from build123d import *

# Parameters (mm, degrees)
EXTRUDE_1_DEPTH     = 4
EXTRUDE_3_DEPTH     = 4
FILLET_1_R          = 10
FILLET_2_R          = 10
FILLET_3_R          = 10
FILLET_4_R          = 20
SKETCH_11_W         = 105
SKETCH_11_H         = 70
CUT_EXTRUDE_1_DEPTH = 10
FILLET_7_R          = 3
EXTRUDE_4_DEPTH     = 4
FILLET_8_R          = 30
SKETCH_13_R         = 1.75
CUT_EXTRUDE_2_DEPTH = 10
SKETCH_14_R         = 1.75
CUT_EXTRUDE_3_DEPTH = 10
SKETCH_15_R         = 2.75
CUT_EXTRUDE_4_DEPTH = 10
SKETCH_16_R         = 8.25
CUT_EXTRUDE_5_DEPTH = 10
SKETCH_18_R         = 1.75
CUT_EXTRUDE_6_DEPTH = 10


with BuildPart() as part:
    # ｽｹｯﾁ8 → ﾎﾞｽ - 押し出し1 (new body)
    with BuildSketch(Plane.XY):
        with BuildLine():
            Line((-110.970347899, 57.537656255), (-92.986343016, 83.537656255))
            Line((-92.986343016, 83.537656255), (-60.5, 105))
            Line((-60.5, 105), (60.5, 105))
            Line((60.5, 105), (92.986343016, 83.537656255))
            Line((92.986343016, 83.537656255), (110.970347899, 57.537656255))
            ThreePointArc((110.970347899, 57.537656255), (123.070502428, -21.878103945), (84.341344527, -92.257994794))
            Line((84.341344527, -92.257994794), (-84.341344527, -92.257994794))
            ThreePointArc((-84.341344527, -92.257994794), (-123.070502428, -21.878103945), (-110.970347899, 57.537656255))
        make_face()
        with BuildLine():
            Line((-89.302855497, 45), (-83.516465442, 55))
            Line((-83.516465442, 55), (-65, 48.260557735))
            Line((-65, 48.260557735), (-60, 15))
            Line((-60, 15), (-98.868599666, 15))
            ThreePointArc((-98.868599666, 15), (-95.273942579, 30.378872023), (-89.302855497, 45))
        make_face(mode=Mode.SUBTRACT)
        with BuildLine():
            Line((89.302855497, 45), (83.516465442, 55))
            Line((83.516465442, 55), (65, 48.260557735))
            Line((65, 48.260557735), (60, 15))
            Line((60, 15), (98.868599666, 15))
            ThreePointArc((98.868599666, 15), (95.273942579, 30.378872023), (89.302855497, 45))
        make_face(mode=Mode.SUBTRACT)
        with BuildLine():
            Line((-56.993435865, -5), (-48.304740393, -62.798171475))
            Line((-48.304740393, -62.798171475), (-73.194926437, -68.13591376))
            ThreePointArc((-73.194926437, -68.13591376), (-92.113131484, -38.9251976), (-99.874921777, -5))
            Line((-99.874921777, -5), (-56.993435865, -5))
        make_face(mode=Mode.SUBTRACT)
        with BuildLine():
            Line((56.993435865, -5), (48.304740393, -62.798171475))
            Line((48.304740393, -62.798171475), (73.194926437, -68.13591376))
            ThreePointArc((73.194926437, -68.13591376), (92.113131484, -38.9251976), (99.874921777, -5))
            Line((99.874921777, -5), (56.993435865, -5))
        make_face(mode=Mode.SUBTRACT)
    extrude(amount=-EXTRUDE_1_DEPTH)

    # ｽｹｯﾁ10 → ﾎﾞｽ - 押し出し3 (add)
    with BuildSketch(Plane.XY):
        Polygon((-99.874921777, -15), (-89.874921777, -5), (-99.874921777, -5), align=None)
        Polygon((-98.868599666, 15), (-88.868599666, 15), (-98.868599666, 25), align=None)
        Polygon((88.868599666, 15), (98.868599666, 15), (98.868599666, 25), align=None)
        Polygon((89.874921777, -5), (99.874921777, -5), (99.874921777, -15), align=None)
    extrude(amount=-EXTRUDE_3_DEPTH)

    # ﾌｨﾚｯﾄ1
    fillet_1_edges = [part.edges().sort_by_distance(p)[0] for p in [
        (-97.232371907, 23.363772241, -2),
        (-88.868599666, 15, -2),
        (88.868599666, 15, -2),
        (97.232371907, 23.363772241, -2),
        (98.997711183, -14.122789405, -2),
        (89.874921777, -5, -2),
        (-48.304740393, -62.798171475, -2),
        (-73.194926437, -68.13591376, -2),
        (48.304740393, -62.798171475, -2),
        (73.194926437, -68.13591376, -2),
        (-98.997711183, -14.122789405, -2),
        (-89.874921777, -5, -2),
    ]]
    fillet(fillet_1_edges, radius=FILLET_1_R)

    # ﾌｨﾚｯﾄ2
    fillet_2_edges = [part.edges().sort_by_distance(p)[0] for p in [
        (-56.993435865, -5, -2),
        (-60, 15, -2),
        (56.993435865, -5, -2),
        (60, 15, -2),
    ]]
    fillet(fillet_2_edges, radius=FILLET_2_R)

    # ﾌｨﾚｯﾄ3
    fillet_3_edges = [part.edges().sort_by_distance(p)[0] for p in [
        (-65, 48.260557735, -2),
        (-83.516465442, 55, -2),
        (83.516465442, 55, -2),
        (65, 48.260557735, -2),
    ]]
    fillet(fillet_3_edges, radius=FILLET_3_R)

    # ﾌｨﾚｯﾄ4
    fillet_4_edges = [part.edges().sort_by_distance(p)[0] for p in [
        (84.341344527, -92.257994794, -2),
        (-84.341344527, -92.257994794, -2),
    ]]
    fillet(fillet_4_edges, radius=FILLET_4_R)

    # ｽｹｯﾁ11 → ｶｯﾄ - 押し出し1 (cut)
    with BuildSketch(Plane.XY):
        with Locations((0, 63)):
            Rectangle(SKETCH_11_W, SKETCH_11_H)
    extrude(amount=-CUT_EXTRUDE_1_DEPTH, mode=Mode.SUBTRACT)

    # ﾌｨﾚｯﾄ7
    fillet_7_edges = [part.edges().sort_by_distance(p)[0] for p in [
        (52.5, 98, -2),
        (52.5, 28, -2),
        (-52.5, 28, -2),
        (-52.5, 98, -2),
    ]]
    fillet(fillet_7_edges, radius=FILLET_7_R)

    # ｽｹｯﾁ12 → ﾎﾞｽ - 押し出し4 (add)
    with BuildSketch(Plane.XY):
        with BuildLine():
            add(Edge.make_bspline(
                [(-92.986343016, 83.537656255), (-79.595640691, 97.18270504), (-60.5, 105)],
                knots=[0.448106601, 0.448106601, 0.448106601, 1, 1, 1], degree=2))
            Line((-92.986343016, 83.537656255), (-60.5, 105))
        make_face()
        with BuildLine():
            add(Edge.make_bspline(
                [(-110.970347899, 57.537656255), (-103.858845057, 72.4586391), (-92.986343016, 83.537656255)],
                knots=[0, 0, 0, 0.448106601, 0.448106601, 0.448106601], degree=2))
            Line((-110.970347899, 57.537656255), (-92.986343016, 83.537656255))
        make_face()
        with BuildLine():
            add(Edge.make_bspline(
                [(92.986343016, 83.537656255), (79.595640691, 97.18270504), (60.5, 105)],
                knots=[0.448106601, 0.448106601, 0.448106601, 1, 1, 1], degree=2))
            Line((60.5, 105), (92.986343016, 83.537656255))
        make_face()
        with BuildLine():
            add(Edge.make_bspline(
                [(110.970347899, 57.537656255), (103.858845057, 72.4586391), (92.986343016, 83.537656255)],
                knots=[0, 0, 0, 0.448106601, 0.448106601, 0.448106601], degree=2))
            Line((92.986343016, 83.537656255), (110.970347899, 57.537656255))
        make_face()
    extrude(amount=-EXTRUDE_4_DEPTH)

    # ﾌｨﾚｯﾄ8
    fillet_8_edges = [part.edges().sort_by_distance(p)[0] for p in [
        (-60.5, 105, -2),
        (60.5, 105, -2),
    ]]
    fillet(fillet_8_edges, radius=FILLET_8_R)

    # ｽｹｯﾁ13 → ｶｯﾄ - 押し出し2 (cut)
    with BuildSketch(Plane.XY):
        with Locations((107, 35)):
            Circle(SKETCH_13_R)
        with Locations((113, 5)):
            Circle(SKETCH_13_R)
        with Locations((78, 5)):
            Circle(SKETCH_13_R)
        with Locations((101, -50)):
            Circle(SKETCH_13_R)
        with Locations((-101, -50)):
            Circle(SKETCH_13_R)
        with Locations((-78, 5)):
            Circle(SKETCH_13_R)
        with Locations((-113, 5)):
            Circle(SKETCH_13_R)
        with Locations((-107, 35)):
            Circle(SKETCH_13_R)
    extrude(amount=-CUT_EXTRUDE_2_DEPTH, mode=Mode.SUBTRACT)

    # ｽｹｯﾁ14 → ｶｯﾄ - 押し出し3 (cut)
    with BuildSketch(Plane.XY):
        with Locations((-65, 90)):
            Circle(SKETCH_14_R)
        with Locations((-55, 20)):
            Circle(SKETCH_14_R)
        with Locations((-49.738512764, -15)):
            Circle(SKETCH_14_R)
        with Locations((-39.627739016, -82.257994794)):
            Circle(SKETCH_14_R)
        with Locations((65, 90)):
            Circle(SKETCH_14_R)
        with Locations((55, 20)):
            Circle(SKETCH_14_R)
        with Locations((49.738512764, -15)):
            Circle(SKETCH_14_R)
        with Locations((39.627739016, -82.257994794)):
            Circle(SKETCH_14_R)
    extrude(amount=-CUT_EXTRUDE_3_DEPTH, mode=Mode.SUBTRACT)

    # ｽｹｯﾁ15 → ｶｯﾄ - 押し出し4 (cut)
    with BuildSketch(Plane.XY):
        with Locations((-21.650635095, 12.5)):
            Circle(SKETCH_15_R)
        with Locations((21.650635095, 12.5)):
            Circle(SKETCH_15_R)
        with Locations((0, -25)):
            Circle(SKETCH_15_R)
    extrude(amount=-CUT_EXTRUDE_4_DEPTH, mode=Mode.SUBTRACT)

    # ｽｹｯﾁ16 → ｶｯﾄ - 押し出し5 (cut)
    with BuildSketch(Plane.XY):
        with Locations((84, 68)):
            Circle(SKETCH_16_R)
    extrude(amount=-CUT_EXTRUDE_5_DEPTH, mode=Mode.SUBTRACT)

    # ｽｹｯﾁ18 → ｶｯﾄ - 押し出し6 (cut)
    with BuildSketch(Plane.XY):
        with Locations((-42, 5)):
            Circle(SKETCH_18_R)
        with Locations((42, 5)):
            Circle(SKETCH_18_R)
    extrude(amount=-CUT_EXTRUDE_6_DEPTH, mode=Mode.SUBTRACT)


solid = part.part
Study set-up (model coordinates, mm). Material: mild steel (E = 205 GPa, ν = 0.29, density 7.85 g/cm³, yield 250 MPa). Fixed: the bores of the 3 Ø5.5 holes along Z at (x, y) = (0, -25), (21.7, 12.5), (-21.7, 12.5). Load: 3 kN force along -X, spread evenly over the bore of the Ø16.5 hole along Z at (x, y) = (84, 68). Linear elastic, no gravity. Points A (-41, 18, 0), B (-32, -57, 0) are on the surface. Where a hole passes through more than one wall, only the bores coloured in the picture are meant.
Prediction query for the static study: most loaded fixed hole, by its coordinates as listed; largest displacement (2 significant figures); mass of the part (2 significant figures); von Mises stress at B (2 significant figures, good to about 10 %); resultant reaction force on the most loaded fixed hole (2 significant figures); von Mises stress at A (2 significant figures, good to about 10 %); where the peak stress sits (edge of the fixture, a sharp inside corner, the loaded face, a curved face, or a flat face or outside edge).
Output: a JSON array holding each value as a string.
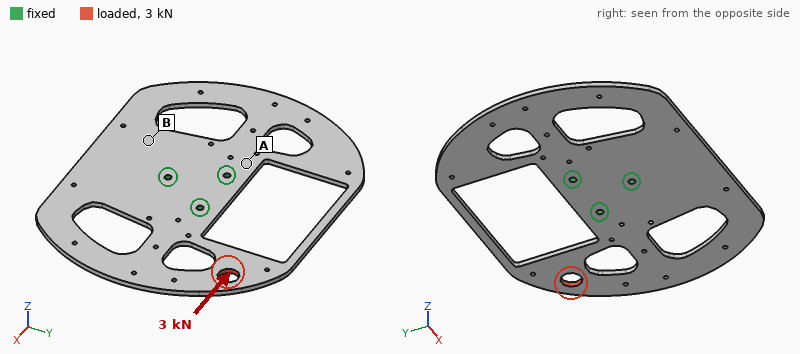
["(21.7, 12.5)", "79 µm", "910 g", "7.8 MPa", "3.6 kN", "18 MPa", "a curved face"]
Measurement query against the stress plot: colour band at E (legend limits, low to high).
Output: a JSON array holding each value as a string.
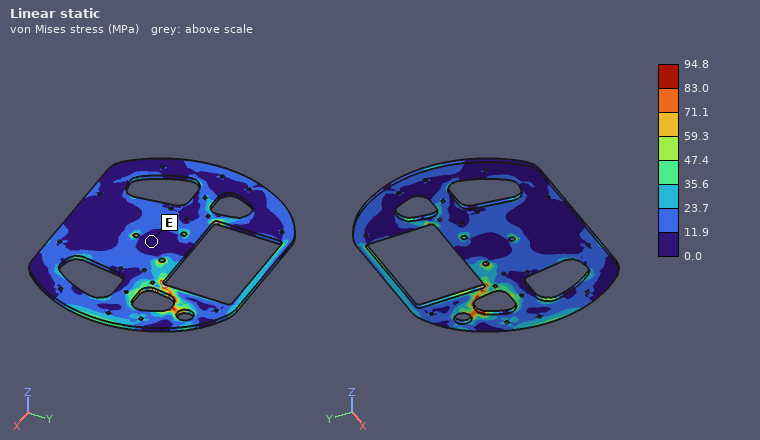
["0.0 to 11.9 MPa"]
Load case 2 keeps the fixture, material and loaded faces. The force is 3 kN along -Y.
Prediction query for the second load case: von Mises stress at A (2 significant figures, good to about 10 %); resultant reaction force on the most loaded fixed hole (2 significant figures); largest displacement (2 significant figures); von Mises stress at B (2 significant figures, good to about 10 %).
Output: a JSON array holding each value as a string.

["7.6 MPa", "4.1 kN", "50 µm", "8.3 MPa"]
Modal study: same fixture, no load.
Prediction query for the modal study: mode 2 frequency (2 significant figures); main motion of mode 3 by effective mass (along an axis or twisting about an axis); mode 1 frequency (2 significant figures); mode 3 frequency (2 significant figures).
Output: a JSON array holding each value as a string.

["230 Hz", "along Z", "220 Hz", "280 Hz"]
